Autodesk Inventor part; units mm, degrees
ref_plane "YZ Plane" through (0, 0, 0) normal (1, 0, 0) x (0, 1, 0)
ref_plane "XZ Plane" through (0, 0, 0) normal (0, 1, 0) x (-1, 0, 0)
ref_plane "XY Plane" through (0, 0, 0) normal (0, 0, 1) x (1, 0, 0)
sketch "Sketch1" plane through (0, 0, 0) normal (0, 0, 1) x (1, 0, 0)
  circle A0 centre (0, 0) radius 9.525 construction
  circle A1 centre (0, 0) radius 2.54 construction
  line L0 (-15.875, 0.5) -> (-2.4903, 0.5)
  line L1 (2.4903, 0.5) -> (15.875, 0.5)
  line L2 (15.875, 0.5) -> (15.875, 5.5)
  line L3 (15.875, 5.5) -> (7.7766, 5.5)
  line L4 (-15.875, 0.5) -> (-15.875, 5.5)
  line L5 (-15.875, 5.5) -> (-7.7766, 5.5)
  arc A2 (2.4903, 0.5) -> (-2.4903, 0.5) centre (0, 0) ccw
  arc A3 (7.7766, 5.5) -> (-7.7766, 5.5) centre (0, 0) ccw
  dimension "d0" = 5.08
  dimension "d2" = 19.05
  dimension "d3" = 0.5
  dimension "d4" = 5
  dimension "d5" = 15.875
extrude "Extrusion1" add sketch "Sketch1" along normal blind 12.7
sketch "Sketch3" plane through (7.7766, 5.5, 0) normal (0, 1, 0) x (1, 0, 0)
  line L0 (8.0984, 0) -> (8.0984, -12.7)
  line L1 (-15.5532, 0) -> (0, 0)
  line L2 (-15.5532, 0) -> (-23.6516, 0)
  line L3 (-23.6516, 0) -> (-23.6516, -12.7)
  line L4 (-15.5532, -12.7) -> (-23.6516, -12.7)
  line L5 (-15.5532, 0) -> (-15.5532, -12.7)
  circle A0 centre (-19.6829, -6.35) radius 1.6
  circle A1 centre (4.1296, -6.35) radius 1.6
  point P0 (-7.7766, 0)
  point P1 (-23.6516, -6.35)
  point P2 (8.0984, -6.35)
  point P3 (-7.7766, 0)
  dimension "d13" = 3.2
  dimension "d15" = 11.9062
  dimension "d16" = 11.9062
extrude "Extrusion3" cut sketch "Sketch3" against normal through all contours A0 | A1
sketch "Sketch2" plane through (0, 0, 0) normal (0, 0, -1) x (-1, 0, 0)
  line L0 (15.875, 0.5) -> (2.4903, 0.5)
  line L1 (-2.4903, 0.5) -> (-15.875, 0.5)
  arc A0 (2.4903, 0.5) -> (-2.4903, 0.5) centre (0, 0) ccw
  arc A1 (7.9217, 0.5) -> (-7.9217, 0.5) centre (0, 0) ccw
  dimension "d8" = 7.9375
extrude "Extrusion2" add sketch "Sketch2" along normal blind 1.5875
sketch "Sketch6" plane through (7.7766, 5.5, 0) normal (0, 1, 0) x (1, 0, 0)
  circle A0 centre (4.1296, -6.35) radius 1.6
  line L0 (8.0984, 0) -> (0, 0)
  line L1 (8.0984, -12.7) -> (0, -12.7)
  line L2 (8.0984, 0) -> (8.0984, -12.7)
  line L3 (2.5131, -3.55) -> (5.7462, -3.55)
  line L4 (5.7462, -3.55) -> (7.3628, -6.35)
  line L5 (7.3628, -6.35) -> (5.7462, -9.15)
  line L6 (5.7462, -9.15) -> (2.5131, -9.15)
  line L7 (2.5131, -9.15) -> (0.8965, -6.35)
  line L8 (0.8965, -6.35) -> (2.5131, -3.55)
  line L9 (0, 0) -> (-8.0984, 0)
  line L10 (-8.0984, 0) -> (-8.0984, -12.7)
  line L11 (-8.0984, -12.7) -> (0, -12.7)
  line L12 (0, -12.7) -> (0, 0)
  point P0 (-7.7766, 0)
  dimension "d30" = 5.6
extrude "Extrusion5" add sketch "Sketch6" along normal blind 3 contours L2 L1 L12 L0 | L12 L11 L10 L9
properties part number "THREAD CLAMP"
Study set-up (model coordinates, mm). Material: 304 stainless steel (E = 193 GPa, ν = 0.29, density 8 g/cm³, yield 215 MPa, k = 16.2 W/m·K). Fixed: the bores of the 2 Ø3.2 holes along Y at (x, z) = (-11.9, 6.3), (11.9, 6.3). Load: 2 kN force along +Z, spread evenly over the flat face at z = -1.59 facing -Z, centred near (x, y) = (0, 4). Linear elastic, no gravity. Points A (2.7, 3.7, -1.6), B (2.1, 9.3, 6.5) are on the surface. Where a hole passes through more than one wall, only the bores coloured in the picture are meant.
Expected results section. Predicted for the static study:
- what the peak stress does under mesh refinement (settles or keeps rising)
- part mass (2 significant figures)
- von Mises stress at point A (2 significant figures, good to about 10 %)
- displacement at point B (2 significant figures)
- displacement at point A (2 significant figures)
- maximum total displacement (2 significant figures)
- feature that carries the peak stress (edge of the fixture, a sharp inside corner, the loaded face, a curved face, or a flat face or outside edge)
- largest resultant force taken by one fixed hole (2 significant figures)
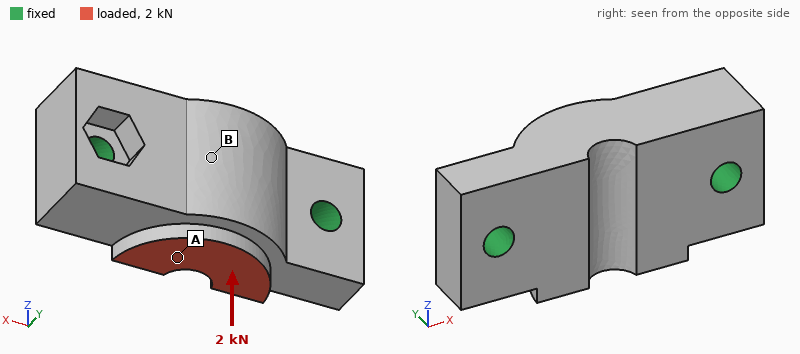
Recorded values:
keeps rising
22 g
34 MPa
3.2 µm
3.1 µm
3.8 µm
edge of the fixture
1.0 kN
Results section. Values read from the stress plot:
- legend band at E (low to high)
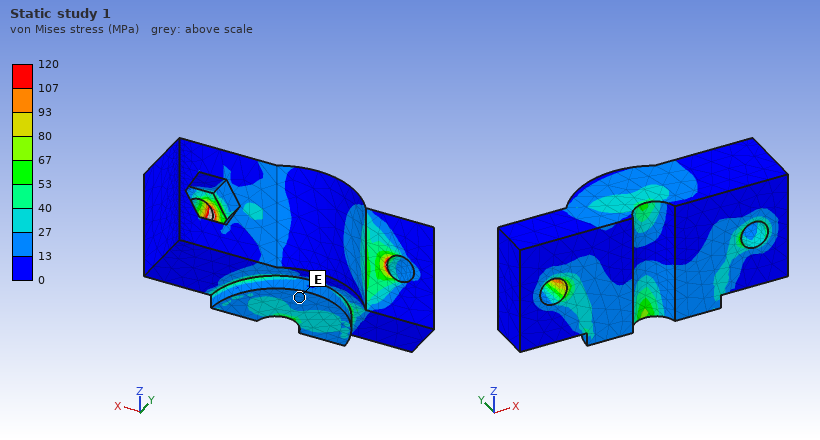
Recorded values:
13 to 27 MPa
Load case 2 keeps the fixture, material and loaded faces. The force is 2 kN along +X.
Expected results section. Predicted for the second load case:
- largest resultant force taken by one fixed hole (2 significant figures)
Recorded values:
1.2 kN
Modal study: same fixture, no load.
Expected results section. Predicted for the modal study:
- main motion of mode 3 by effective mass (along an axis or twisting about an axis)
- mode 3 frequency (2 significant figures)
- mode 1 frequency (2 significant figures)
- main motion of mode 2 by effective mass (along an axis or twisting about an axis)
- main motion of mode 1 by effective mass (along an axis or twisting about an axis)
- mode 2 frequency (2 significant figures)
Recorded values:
along Z
45 kHz
28 kHz
along Y
along Z
34 kHz
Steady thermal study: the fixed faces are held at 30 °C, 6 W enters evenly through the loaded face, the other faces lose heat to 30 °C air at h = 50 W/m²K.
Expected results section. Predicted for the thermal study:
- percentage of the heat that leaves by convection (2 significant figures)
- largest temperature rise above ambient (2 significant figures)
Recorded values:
12 %
38 K
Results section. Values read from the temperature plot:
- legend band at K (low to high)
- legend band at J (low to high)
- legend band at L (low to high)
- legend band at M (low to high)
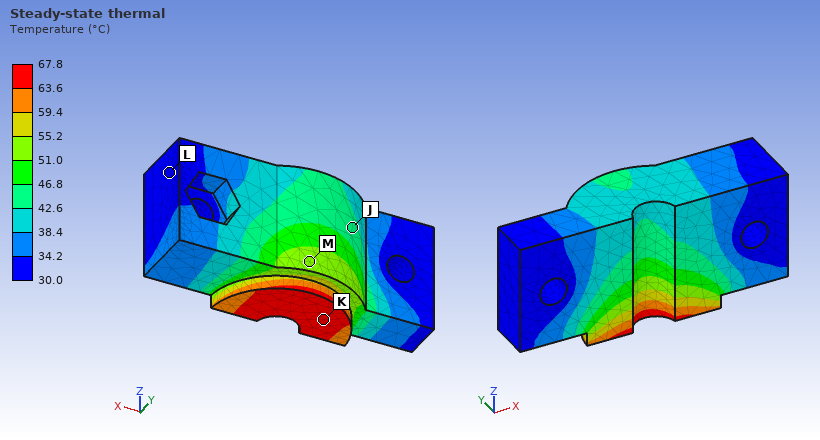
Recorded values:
63.6 to 67.8 °C
42.6 to 46.8 °C
30.0 to 34.2 °C
51.0 to 55.2 °C
